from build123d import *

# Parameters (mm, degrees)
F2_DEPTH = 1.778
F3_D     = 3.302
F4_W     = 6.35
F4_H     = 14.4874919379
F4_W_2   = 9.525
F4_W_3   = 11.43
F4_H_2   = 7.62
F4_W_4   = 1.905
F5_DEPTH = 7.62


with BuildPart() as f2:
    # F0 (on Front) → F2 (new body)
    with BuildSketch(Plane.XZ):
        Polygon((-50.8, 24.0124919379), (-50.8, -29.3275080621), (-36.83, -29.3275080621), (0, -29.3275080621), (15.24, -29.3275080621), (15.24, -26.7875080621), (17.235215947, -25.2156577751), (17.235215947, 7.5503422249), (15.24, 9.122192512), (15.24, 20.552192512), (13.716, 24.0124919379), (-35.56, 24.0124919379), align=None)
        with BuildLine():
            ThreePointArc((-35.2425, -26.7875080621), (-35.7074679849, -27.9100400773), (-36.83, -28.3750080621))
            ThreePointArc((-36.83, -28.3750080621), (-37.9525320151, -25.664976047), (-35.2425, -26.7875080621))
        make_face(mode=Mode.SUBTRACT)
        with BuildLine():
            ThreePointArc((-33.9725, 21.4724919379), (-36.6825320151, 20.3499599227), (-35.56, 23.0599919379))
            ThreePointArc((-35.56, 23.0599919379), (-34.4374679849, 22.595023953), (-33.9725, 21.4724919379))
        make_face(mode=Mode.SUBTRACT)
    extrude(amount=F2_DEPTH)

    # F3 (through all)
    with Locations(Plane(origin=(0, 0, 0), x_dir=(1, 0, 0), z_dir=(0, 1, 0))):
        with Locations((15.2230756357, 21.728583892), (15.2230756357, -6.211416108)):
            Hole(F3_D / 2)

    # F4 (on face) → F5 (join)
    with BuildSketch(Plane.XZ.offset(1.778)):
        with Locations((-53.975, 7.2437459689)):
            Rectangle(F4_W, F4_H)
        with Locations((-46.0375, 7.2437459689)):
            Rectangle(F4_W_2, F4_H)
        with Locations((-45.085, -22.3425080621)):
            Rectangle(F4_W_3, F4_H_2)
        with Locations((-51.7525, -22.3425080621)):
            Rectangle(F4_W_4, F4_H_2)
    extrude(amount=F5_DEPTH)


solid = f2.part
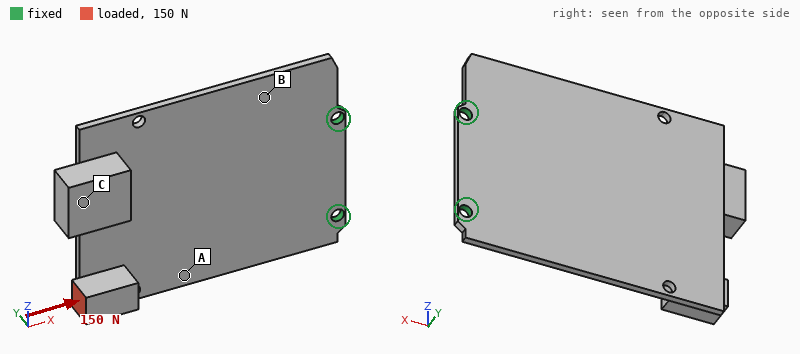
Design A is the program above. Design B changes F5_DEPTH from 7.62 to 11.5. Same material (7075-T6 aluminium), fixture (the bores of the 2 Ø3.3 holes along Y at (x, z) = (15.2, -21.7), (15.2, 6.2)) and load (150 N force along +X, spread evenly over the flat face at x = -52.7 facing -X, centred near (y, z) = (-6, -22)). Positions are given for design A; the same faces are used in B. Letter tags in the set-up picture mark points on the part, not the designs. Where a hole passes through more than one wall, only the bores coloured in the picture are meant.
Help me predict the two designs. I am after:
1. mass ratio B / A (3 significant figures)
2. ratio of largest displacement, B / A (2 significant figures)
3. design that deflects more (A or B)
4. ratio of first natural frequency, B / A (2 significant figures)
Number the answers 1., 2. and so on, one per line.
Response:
1. 1.15
2. 1.4
3. B
4. 0.87
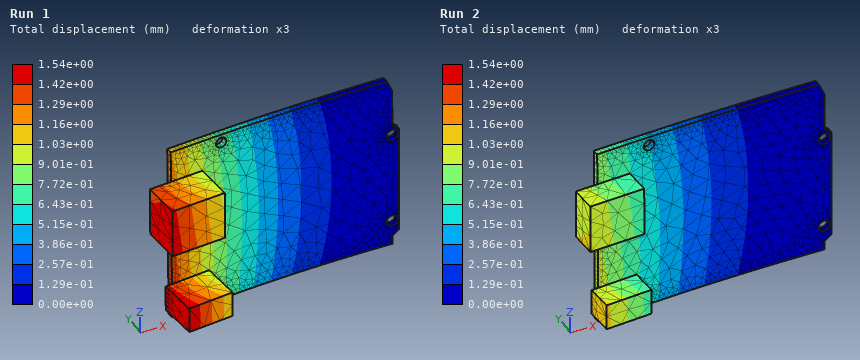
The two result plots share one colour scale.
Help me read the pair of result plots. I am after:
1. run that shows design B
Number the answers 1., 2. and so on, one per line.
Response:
1. Run 1
